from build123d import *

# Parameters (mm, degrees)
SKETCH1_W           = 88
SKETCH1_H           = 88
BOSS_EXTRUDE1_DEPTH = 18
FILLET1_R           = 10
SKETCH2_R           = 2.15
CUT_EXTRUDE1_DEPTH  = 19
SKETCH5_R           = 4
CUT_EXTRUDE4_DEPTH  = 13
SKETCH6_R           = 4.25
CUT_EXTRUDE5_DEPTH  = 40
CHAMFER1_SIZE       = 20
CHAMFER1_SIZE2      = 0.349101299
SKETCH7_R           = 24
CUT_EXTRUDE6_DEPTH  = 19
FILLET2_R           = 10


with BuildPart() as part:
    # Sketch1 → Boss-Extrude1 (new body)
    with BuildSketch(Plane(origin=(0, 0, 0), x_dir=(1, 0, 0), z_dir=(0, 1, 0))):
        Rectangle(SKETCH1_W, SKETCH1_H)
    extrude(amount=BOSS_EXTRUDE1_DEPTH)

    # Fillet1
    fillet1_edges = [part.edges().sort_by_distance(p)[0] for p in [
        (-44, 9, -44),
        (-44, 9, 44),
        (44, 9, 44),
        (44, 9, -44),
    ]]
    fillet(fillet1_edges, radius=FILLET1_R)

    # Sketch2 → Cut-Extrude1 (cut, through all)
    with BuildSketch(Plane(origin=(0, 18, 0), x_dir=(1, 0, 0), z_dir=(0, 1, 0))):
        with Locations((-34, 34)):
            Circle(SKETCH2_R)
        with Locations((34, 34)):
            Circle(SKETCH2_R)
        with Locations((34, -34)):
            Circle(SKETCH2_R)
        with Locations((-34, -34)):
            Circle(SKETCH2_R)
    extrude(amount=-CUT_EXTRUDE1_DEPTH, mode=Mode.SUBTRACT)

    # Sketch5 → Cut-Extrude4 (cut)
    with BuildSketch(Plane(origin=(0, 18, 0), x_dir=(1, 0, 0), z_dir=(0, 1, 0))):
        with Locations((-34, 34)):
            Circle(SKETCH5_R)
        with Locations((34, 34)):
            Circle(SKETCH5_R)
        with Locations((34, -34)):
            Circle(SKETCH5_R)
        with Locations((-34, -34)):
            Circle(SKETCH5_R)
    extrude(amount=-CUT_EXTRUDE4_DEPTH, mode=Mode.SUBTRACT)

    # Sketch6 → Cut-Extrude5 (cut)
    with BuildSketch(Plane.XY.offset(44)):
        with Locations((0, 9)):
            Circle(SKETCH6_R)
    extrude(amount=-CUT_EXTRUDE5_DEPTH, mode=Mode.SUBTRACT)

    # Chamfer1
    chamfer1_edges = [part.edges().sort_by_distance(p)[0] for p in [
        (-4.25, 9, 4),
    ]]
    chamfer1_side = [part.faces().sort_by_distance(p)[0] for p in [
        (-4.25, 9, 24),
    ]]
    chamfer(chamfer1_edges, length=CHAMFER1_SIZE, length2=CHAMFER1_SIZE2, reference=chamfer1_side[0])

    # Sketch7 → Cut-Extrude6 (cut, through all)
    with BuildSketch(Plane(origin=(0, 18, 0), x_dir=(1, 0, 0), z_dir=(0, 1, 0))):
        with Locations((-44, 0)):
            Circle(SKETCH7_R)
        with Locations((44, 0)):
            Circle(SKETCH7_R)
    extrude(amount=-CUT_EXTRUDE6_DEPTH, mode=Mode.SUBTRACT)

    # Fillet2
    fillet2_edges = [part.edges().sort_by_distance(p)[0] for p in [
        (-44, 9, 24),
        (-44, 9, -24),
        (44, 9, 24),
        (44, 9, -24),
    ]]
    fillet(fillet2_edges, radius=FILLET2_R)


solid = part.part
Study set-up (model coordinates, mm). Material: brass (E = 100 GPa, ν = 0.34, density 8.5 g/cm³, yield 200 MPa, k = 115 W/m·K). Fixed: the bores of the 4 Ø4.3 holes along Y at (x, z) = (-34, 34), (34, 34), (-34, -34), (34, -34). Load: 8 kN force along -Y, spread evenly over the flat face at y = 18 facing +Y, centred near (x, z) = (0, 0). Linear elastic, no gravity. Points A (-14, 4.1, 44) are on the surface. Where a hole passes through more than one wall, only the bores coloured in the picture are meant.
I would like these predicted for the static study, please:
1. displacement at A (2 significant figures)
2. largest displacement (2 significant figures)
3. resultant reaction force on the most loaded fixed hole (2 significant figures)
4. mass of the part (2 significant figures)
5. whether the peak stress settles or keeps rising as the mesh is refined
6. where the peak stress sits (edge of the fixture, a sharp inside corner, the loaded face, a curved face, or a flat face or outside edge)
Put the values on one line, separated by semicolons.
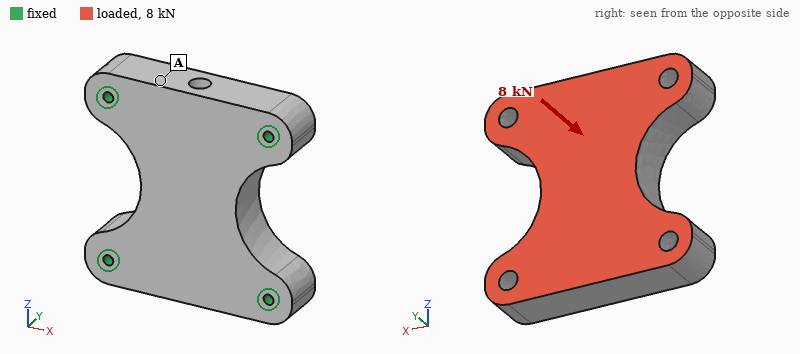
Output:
6.5 µm; 13 µm; 2.4 kN; 840 g; keeps rising; edge of the fixture
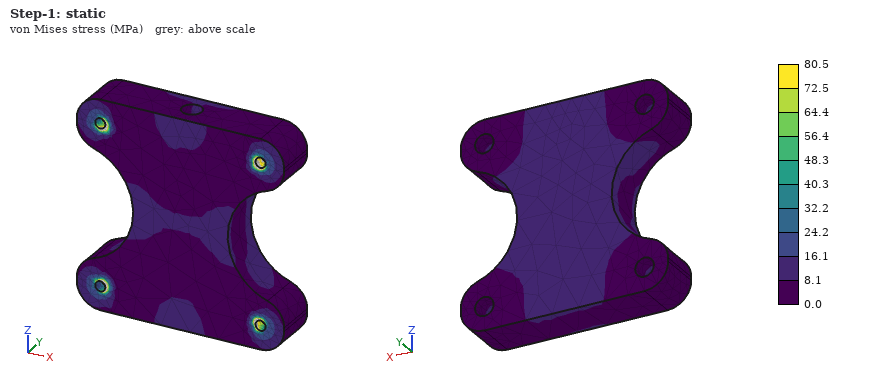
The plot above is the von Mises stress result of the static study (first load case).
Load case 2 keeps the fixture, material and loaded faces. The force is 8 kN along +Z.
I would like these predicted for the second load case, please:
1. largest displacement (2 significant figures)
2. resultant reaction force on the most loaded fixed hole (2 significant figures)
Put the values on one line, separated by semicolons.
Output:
12 µm; 2.4 kN
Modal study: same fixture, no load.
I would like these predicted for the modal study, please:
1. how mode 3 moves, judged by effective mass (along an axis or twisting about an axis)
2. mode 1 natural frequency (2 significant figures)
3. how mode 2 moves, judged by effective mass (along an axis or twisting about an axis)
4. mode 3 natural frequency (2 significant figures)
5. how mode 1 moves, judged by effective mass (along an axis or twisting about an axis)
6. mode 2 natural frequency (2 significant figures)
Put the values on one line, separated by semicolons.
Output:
along Z; 4900 Hz; along Z; 7200 Hz; along Y; 6500 Hz
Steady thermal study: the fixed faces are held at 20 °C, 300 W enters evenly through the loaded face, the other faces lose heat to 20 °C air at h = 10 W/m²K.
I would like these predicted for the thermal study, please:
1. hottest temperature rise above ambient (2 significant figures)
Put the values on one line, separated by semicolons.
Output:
56 K
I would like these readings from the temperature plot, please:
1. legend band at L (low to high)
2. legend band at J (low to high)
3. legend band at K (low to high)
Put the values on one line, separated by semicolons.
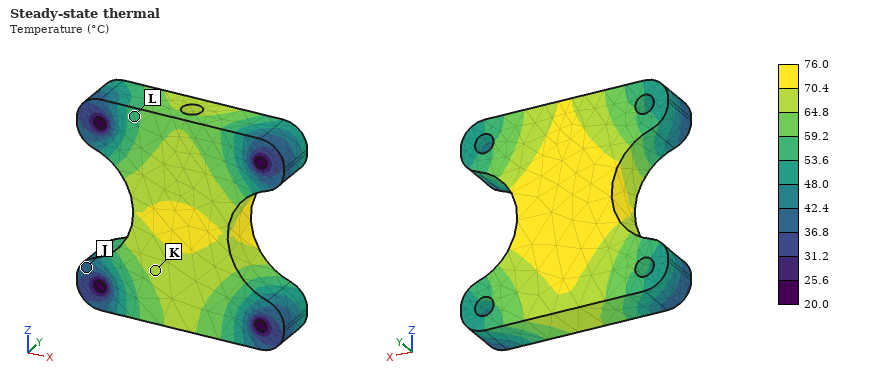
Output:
53.6 to 59.2 °C; 36.8 to 42.4 °C; 64.8 to 70.4 °C
